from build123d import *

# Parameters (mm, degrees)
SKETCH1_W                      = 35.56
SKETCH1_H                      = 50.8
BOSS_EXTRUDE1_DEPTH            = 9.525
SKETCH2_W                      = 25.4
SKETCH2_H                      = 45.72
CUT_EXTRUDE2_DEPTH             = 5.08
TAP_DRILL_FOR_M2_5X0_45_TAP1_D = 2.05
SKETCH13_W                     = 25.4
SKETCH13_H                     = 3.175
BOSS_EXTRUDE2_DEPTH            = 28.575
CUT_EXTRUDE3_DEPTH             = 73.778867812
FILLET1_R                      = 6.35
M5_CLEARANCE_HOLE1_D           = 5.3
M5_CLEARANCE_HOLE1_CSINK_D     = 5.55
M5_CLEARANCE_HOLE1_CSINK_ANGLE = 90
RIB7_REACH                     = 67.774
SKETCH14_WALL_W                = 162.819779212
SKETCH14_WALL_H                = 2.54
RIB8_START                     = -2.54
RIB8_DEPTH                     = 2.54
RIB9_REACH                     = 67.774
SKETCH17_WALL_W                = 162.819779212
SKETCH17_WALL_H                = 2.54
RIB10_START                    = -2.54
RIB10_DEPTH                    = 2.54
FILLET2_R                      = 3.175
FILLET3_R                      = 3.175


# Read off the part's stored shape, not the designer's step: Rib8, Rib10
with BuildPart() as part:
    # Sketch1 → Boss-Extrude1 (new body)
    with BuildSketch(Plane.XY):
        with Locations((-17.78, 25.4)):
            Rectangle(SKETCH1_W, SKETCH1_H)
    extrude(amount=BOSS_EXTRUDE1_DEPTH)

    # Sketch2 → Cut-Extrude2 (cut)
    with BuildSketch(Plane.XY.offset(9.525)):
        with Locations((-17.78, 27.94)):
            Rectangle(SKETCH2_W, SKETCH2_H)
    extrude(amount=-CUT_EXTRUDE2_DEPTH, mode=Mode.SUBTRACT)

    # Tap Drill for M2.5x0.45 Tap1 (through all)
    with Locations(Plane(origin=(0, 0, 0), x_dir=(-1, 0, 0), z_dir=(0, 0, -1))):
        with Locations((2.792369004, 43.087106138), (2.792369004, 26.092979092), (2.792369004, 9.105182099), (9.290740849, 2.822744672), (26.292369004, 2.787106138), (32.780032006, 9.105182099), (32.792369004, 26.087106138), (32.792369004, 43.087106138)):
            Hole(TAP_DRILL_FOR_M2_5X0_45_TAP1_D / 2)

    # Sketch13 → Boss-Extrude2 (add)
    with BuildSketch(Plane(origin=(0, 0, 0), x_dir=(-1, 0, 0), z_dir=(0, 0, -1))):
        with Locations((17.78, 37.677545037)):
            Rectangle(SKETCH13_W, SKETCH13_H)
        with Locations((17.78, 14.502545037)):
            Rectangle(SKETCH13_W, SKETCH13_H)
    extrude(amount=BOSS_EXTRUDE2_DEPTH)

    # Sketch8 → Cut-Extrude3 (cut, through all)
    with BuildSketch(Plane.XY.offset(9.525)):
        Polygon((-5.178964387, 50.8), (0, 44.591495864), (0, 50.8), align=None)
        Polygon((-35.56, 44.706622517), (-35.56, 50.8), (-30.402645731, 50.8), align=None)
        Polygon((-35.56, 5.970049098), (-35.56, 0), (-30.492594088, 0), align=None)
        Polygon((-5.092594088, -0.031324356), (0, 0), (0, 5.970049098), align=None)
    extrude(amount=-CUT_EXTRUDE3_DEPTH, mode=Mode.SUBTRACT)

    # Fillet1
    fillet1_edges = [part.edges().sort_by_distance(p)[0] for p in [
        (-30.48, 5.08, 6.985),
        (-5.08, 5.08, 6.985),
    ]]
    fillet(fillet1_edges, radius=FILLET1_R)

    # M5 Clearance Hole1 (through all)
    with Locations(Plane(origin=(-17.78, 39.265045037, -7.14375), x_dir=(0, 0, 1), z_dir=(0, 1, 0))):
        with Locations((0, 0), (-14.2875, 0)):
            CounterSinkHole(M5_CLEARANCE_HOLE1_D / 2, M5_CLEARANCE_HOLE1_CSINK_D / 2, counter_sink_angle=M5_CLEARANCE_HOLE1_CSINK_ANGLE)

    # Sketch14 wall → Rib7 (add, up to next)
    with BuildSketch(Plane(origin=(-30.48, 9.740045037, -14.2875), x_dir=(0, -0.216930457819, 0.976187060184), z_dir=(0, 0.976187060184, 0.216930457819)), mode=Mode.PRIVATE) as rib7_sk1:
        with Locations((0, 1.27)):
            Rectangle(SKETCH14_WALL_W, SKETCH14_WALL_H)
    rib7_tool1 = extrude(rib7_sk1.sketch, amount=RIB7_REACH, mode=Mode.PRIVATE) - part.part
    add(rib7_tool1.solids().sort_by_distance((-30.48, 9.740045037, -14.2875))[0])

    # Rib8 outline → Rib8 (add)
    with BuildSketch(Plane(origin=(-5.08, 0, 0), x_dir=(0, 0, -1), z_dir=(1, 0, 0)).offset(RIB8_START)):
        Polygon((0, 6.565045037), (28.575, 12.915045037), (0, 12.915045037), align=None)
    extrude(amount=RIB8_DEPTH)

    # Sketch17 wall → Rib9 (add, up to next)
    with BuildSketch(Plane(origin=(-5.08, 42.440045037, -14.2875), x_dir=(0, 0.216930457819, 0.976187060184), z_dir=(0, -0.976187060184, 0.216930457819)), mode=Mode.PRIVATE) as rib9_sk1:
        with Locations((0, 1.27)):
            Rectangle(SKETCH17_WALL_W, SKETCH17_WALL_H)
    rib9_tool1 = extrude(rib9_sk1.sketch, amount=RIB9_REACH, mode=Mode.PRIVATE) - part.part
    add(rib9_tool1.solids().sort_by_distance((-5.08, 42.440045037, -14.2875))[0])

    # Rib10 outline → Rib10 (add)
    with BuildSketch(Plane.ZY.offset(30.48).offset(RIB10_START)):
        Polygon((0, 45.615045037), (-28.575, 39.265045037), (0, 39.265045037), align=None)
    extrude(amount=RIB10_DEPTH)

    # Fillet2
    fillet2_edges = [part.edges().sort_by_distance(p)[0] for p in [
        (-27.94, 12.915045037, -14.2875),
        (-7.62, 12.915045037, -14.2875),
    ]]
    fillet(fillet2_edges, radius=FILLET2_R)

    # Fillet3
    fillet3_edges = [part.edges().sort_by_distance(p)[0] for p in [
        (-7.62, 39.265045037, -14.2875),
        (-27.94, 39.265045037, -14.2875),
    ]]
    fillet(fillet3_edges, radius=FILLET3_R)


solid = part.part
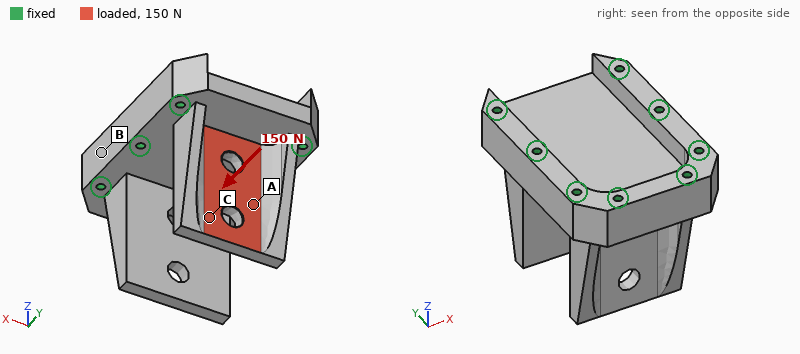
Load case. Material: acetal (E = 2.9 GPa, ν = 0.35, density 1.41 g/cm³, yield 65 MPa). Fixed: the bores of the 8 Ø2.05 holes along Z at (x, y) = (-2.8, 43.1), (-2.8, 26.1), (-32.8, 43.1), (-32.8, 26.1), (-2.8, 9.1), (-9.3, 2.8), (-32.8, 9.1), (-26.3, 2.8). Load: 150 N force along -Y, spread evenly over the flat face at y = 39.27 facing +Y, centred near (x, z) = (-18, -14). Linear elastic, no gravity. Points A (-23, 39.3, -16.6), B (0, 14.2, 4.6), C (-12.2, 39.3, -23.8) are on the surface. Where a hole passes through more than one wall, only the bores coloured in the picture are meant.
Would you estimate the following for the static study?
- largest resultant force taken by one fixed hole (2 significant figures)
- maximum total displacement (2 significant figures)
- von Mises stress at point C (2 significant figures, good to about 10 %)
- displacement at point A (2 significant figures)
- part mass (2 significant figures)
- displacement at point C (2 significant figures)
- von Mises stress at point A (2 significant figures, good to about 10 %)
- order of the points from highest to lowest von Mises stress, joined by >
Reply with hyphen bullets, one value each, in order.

- 75 N
- 0.68 mm
- 3.6 MPa
- 0.31 mm
- 23 g
- 0.50 mm
- 5.0 MPa
- A > C > B
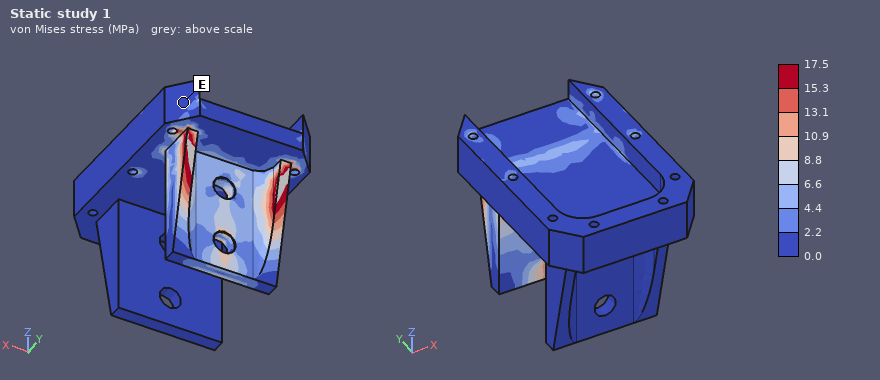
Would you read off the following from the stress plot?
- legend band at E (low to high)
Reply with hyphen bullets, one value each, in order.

- 0.0 to 2.2 MPa
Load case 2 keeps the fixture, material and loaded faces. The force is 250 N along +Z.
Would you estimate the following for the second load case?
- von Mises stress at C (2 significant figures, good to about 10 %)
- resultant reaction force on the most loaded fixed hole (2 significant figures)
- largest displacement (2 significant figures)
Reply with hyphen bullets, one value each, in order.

- 3.3 MPa
- 100 N
- 69 µm
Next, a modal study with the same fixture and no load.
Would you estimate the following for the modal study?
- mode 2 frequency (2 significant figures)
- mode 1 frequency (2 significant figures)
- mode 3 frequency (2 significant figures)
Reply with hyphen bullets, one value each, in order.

- 1700 Hz
- 1700 Hz
- 2800 Hz
